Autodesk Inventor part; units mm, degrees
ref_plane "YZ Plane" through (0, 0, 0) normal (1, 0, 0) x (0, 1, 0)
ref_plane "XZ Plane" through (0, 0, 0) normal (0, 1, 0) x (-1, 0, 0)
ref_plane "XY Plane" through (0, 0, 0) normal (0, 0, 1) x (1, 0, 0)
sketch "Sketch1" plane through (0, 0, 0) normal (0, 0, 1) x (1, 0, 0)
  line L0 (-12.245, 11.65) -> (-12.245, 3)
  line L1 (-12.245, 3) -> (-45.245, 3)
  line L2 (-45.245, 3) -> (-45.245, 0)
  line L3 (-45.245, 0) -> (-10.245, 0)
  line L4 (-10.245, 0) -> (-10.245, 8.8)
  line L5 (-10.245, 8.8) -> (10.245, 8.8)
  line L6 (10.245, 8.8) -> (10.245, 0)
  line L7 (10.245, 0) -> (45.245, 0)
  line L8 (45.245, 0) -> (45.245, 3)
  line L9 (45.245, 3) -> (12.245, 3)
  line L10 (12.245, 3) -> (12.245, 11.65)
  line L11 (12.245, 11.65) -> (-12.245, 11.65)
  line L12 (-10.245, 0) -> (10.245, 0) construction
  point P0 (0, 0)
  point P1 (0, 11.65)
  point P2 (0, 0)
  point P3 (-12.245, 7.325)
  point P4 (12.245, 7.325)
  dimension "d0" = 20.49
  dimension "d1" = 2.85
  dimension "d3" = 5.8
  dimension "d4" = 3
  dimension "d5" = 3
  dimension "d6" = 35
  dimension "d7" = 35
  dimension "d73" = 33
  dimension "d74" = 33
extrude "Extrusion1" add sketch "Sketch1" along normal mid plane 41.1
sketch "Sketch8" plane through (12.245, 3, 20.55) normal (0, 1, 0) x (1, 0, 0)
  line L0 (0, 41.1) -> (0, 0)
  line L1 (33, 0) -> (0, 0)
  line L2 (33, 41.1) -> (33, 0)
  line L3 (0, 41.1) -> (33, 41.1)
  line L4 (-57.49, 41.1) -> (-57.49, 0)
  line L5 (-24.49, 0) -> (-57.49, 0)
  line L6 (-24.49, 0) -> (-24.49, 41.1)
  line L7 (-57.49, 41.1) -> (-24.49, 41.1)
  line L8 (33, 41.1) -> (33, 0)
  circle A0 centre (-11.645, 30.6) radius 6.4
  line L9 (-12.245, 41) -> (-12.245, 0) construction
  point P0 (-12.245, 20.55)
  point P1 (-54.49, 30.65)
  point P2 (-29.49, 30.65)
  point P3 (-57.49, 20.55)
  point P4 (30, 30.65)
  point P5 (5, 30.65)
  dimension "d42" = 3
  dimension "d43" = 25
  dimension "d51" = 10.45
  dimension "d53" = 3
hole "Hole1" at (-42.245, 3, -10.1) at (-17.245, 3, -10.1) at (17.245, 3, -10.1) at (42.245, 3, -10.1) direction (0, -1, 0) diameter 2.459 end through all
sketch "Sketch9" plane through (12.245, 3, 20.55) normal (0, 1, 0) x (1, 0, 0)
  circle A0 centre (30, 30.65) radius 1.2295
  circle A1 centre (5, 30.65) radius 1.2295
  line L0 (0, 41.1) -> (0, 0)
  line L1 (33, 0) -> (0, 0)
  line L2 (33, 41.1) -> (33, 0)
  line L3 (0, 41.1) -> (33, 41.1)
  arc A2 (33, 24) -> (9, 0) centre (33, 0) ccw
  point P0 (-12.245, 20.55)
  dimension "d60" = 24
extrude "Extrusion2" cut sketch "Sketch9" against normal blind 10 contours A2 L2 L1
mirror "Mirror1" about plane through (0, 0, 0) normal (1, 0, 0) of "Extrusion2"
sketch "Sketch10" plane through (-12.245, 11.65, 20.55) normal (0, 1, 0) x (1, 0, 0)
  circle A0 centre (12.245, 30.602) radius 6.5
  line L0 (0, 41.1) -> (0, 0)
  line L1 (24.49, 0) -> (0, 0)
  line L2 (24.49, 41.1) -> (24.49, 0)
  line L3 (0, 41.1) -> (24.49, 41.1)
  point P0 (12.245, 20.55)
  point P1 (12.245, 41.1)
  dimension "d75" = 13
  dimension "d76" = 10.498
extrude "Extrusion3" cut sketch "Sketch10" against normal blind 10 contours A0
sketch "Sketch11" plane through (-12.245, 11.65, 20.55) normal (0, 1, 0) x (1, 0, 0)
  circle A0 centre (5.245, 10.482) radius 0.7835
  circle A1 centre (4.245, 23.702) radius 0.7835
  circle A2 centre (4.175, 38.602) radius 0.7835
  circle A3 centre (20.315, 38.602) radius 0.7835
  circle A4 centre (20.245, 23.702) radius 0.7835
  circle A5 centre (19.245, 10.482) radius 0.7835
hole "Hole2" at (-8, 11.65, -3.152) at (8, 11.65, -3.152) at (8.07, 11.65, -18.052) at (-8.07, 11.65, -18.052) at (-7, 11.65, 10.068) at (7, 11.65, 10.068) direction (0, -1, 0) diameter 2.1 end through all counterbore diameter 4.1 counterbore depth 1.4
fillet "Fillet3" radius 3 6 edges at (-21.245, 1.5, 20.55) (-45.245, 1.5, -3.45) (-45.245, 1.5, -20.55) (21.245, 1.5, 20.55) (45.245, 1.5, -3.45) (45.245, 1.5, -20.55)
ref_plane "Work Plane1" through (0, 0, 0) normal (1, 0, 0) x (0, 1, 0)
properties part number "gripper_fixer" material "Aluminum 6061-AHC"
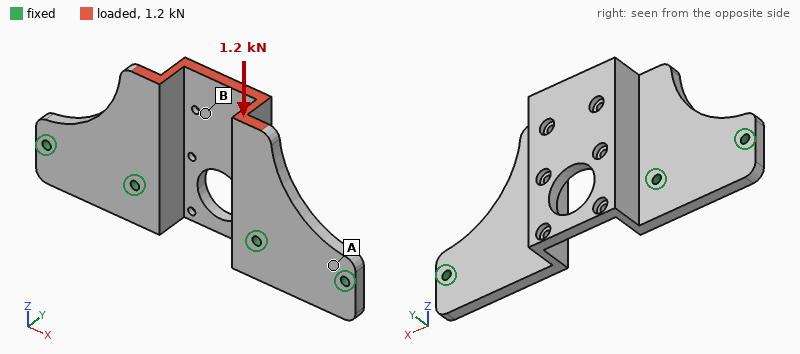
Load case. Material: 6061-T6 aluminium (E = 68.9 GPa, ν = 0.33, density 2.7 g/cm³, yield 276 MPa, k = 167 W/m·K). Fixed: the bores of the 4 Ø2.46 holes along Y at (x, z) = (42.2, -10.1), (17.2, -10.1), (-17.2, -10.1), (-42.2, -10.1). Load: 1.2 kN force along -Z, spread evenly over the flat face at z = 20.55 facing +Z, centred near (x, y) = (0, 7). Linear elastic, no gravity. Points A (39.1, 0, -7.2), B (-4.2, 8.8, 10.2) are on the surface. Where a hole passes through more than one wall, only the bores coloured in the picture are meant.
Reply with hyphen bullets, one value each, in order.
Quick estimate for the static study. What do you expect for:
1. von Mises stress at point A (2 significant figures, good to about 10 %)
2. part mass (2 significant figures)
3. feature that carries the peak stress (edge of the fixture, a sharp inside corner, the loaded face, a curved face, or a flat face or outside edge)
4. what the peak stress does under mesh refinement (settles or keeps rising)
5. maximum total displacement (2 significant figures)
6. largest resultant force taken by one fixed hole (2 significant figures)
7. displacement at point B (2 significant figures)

- 20 MPa
- 25 g
- edge of the fixture
- keeps rising
- 0.13 mm
- 720 N
- 0.087 mm
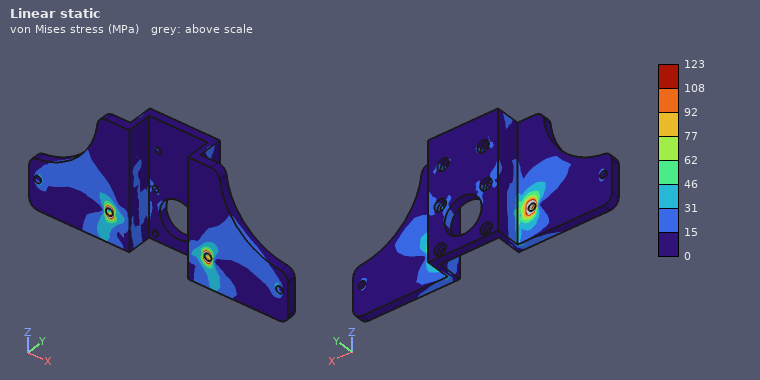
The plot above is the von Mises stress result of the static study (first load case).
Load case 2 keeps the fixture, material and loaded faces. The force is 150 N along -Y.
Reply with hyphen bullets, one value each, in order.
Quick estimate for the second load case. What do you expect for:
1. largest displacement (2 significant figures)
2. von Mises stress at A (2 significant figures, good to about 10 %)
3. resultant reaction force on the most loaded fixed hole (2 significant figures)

- 0.10 mm
- 14 MPa
- 96 N
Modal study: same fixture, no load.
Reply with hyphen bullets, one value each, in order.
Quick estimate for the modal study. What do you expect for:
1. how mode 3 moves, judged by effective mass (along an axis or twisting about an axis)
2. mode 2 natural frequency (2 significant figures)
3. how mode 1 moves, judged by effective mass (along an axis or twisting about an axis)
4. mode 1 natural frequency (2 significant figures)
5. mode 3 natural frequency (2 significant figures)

- along X
- 6700 Hz
- along Y
- 2900 Hz
- 9500 Hz
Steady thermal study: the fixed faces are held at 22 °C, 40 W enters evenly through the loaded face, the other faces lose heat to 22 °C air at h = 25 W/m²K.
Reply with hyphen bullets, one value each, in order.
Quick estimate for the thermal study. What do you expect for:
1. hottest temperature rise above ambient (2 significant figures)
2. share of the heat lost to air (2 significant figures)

- 56 K
- 8.8 %
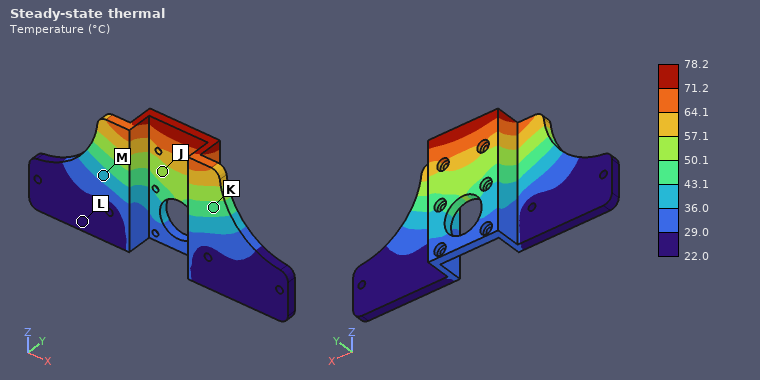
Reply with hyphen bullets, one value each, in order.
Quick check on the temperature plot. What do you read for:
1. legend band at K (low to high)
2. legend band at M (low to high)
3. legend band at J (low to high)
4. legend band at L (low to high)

- 43.1 to 50.1 °C
- 36.0 to 43.1 °C
- 50.1 to 57.1 °C
- 22.0 to 29.0 °C
